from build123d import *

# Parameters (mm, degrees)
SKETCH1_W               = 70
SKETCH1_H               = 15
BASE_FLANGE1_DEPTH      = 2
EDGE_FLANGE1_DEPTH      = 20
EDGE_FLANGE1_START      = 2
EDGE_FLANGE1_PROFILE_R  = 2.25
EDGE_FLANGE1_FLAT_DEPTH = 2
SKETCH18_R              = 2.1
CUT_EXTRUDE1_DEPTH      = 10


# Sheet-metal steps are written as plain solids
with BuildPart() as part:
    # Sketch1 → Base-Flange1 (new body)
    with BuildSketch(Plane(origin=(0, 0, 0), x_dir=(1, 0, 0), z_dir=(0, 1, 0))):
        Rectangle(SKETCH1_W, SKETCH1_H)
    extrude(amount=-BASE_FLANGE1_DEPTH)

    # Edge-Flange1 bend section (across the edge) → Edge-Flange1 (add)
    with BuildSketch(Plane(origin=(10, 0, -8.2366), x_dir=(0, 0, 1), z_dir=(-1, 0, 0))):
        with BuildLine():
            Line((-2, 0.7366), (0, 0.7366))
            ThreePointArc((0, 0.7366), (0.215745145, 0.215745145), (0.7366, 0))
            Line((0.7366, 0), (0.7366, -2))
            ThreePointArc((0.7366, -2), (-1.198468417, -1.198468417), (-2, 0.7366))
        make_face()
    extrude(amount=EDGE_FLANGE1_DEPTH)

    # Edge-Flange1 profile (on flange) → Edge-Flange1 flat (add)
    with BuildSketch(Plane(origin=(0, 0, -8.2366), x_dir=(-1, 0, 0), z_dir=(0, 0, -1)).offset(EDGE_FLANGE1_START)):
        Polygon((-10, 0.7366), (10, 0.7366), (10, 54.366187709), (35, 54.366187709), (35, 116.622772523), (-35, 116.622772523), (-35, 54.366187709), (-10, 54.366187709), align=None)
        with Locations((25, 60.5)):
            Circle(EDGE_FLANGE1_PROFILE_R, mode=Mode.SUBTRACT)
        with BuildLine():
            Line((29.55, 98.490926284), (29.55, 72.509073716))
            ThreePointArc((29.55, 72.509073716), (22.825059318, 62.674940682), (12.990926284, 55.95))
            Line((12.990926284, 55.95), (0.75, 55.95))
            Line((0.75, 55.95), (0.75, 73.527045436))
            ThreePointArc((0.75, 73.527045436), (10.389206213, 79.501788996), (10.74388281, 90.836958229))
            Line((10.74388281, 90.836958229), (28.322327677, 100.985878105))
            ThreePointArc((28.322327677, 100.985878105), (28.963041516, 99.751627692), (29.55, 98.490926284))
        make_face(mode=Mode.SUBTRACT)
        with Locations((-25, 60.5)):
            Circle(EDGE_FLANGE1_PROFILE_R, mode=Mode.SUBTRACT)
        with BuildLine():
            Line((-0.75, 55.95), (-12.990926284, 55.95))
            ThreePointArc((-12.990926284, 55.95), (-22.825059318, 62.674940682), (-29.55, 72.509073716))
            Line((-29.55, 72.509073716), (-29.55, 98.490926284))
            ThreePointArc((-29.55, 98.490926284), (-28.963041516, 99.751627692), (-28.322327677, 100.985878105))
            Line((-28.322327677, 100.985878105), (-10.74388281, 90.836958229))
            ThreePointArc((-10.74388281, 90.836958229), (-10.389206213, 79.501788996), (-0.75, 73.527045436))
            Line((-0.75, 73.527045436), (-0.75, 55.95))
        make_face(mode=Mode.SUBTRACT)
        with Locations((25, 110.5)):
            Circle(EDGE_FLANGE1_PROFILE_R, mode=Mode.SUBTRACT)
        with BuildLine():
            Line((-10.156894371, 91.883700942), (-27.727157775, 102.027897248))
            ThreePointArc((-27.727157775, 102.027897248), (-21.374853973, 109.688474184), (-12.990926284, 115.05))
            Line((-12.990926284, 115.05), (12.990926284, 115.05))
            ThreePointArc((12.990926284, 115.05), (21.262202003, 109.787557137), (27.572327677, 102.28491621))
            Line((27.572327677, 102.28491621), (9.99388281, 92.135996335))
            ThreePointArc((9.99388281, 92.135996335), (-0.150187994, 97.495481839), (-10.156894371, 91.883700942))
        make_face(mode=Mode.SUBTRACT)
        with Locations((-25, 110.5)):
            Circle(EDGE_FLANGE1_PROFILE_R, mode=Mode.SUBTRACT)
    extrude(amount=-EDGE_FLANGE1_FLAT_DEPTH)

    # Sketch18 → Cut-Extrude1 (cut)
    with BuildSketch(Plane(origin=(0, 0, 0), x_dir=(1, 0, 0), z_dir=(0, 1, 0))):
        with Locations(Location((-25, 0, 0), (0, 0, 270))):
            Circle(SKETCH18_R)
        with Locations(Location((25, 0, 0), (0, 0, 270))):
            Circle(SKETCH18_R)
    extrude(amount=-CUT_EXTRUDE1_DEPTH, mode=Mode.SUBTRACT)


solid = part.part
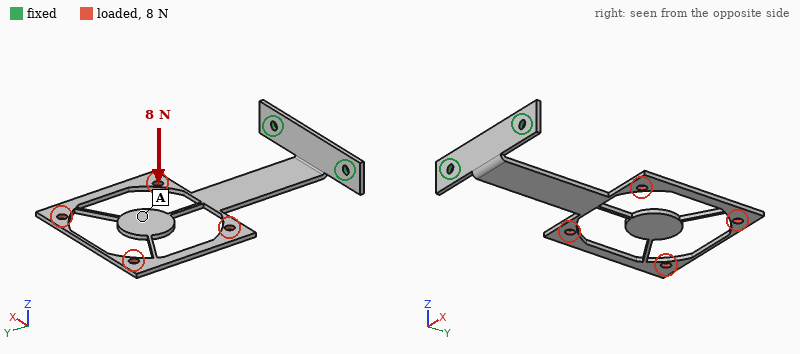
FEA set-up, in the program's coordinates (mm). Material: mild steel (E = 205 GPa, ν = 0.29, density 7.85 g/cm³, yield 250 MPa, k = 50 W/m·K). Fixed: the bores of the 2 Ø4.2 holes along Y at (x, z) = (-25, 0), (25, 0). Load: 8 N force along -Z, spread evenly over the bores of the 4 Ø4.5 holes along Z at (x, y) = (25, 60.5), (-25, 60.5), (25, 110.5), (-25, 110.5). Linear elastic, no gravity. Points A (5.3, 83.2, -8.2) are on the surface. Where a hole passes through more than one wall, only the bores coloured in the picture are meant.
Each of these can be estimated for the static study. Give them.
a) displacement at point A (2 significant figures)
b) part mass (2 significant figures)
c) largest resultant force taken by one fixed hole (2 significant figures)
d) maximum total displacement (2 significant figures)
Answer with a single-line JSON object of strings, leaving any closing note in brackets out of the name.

{"displacement at point A": "0.94 mm", "part mass": "61 g", "largest resultant force taken by one fixed hole": "4.1 N", "maximum total displacement": "1.6 mm"}
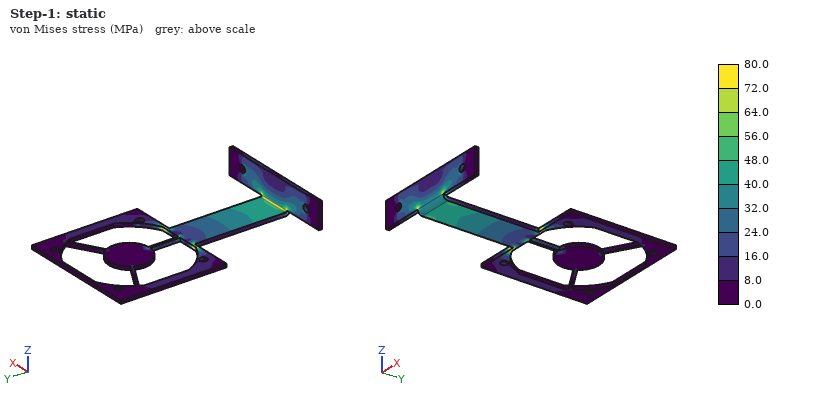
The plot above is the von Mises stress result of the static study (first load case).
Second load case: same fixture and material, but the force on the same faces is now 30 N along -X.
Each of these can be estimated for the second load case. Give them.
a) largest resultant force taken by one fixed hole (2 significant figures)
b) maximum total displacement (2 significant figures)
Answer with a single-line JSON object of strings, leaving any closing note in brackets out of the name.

{"largest resultant force taken by one fixed hole": "78 N", "maximum total displacement": "0.72 mm"}
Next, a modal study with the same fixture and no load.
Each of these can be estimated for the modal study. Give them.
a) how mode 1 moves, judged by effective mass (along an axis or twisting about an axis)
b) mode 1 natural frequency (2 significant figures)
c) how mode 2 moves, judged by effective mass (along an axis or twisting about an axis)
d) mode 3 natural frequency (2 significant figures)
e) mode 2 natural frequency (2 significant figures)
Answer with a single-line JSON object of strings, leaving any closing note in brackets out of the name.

{"how mode 1 moves, judged by effective mass": "along Z", "mode 1 natural frequency": "80 Hz", "how mode 2 moves, judged by effective mass": "along X", "mode 3 natural frequency": "230 Hz", "mode 2 natural frequency": "220 Hz"}
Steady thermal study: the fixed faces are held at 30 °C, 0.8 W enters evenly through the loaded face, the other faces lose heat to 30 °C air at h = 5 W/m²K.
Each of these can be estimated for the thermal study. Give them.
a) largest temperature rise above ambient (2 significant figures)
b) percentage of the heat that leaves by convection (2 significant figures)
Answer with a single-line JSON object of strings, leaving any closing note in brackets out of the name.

{"largest temperature rise above ambient": "25 K", "percentage of the heat that leaves by convection": "68 %"}
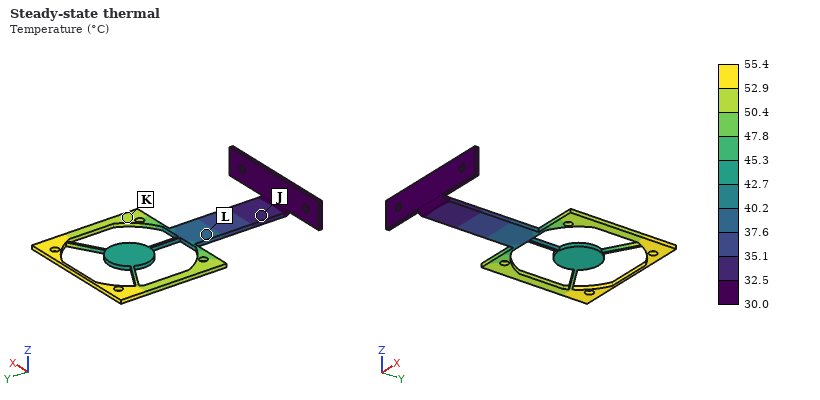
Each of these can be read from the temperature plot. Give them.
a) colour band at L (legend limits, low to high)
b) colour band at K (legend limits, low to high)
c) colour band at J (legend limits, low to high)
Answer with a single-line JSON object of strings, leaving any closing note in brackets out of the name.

{"colour band at L": "37.6 to 40.2 °C", "colour band at K": "50.4 to 52.9 °C", "colour band at J": "32.5 to 35.1 °C"}
